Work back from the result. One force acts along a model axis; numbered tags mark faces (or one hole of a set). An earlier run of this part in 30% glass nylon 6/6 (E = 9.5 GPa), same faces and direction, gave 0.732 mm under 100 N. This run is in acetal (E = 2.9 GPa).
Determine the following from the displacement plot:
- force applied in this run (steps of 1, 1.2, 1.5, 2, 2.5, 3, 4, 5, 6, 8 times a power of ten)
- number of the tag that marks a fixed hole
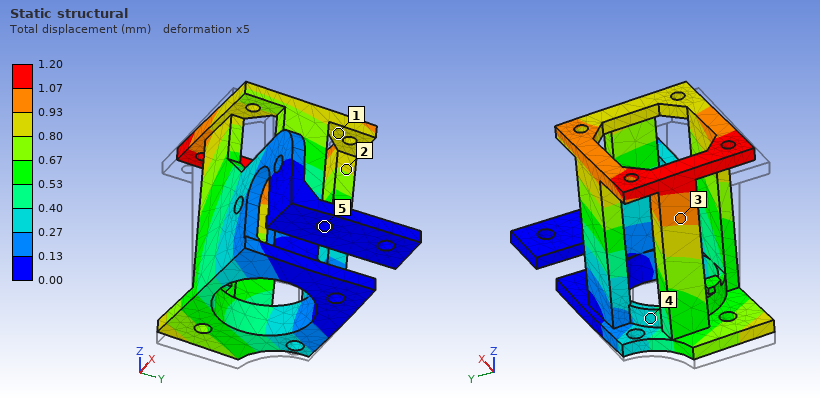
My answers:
50 N
5
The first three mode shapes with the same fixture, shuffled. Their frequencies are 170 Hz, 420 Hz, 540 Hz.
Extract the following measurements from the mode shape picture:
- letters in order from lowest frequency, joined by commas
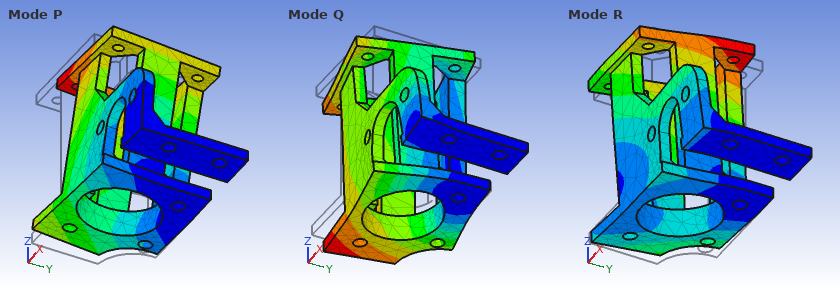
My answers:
P, R, Q
